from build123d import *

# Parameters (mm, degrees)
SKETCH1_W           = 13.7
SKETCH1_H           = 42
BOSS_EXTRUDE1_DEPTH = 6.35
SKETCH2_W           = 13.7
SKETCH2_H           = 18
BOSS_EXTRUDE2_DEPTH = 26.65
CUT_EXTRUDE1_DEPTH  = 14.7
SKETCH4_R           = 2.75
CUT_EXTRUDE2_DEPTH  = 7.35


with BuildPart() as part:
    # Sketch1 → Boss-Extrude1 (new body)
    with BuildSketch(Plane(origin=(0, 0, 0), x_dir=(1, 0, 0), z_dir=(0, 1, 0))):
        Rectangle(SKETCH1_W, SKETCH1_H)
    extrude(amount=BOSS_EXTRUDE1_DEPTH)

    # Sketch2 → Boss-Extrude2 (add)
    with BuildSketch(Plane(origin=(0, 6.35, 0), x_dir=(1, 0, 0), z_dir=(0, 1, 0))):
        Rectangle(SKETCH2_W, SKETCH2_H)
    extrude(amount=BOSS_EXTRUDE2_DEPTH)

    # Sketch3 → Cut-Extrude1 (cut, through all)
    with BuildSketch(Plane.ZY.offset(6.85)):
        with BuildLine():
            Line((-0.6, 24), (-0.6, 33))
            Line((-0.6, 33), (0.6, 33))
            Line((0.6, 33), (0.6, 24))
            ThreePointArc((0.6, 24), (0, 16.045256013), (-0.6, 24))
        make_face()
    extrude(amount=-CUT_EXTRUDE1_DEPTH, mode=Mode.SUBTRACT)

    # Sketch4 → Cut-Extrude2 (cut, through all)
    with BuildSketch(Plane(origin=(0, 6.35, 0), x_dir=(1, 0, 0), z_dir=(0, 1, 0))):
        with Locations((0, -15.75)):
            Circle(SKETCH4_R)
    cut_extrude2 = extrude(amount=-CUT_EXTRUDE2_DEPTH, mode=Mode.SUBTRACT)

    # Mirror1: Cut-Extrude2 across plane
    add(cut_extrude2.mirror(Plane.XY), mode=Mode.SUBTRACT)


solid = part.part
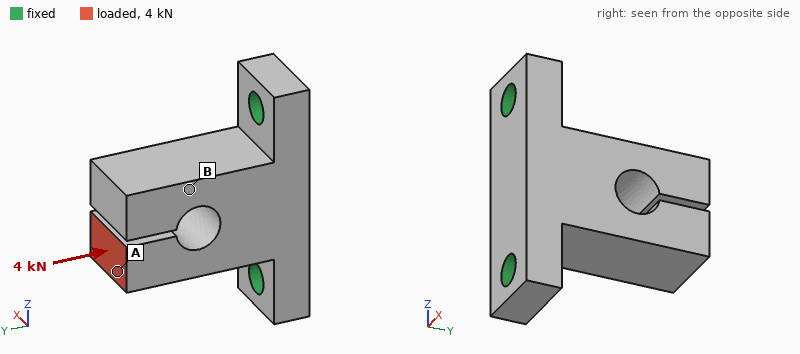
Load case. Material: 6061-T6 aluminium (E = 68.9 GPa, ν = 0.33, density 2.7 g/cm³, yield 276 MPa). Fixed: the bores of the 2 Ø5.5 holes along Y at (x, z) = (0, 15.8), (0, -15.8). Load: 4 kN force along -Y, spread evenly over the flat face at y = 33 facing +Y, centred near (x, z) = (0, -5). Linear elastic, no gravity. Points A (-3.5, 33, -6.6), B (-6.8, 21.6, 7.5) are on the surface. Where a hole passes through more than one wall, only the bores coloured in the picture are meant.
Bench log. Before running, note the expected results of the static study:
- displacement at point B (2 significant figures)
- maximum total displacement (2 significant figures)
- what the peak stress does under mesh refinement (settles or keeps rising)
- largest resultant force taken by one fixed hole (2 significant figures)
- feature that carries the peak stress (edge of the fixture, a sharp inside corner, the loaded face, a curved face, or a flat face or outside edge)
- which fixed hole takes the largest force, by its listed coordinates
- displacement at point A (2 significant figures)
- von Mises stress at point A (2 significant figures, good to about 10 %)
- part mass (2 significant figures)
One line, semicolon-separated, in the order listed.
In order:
13 µm; 65 µm; keeps rising; 2.9 kN; edge of the fixture; (0, -15.8); 48 µm; 35 MPa; 25 g
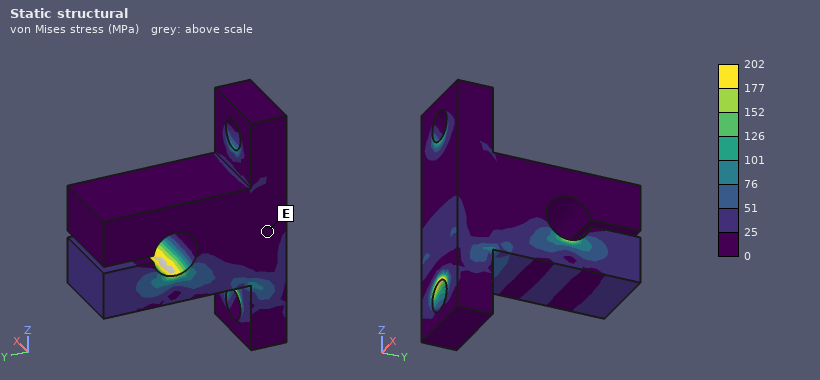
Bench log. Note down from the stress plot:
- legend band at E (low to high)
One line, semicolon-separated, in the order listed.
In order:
0 to 25 MPa
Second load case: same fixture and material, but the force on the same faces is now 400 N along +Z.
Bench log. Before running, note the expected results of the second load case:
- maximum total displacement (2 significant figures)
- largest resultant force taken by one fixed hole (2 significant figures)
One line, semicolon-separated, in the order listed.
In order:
84 µm; 580 N
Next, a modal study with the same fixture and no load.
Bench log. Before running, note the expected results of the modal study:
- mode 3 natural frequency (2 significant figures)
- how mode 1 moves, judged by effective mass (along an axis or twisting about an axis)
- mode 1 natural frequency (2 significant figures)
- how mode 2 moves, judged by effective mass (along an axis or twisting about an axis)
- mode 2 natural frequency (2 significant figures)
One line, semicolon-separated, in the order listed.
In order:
9400 Hz; along X; 5200 Hz; along Z; 7900 Hz
